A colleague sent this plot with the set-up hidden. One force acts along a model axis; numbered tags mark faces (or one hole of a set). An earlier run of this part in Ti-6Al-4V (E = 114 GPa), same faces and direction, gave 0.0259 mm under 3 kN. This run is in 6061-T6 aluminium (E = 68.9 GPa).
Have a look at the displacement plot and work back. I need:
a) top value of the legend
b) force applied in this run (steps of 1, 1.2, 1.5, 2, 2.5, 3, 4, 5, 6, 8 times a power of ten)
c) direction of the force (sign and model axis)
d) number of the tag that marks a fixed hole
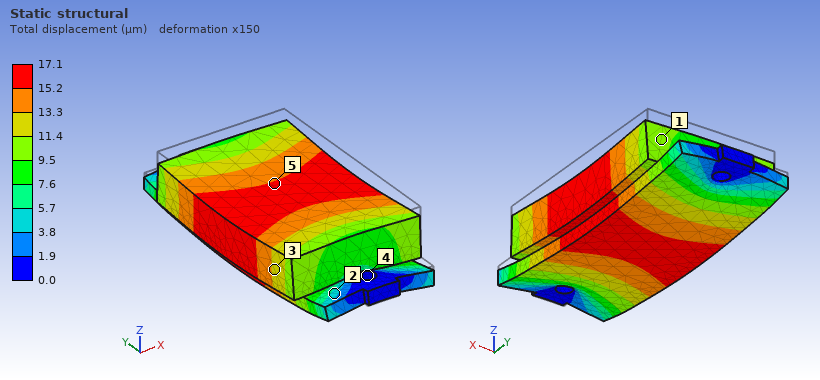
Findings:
17.1 µm
1.2 kN
-Z
4
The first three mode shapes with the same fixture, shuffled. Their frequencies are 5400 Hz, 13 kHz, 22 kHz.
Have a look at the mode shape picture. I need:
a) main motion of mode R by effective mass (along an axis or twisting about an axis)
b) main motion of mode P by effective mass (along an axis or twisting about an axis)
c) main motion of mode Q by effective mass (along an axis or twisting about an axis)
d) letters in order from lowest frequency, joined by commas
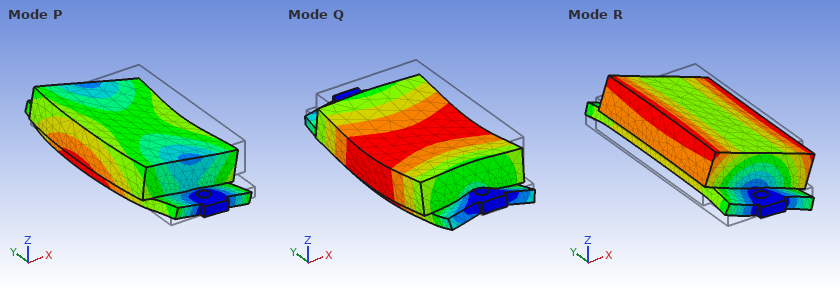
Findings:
along X
along X
along Z
R, Q, P
